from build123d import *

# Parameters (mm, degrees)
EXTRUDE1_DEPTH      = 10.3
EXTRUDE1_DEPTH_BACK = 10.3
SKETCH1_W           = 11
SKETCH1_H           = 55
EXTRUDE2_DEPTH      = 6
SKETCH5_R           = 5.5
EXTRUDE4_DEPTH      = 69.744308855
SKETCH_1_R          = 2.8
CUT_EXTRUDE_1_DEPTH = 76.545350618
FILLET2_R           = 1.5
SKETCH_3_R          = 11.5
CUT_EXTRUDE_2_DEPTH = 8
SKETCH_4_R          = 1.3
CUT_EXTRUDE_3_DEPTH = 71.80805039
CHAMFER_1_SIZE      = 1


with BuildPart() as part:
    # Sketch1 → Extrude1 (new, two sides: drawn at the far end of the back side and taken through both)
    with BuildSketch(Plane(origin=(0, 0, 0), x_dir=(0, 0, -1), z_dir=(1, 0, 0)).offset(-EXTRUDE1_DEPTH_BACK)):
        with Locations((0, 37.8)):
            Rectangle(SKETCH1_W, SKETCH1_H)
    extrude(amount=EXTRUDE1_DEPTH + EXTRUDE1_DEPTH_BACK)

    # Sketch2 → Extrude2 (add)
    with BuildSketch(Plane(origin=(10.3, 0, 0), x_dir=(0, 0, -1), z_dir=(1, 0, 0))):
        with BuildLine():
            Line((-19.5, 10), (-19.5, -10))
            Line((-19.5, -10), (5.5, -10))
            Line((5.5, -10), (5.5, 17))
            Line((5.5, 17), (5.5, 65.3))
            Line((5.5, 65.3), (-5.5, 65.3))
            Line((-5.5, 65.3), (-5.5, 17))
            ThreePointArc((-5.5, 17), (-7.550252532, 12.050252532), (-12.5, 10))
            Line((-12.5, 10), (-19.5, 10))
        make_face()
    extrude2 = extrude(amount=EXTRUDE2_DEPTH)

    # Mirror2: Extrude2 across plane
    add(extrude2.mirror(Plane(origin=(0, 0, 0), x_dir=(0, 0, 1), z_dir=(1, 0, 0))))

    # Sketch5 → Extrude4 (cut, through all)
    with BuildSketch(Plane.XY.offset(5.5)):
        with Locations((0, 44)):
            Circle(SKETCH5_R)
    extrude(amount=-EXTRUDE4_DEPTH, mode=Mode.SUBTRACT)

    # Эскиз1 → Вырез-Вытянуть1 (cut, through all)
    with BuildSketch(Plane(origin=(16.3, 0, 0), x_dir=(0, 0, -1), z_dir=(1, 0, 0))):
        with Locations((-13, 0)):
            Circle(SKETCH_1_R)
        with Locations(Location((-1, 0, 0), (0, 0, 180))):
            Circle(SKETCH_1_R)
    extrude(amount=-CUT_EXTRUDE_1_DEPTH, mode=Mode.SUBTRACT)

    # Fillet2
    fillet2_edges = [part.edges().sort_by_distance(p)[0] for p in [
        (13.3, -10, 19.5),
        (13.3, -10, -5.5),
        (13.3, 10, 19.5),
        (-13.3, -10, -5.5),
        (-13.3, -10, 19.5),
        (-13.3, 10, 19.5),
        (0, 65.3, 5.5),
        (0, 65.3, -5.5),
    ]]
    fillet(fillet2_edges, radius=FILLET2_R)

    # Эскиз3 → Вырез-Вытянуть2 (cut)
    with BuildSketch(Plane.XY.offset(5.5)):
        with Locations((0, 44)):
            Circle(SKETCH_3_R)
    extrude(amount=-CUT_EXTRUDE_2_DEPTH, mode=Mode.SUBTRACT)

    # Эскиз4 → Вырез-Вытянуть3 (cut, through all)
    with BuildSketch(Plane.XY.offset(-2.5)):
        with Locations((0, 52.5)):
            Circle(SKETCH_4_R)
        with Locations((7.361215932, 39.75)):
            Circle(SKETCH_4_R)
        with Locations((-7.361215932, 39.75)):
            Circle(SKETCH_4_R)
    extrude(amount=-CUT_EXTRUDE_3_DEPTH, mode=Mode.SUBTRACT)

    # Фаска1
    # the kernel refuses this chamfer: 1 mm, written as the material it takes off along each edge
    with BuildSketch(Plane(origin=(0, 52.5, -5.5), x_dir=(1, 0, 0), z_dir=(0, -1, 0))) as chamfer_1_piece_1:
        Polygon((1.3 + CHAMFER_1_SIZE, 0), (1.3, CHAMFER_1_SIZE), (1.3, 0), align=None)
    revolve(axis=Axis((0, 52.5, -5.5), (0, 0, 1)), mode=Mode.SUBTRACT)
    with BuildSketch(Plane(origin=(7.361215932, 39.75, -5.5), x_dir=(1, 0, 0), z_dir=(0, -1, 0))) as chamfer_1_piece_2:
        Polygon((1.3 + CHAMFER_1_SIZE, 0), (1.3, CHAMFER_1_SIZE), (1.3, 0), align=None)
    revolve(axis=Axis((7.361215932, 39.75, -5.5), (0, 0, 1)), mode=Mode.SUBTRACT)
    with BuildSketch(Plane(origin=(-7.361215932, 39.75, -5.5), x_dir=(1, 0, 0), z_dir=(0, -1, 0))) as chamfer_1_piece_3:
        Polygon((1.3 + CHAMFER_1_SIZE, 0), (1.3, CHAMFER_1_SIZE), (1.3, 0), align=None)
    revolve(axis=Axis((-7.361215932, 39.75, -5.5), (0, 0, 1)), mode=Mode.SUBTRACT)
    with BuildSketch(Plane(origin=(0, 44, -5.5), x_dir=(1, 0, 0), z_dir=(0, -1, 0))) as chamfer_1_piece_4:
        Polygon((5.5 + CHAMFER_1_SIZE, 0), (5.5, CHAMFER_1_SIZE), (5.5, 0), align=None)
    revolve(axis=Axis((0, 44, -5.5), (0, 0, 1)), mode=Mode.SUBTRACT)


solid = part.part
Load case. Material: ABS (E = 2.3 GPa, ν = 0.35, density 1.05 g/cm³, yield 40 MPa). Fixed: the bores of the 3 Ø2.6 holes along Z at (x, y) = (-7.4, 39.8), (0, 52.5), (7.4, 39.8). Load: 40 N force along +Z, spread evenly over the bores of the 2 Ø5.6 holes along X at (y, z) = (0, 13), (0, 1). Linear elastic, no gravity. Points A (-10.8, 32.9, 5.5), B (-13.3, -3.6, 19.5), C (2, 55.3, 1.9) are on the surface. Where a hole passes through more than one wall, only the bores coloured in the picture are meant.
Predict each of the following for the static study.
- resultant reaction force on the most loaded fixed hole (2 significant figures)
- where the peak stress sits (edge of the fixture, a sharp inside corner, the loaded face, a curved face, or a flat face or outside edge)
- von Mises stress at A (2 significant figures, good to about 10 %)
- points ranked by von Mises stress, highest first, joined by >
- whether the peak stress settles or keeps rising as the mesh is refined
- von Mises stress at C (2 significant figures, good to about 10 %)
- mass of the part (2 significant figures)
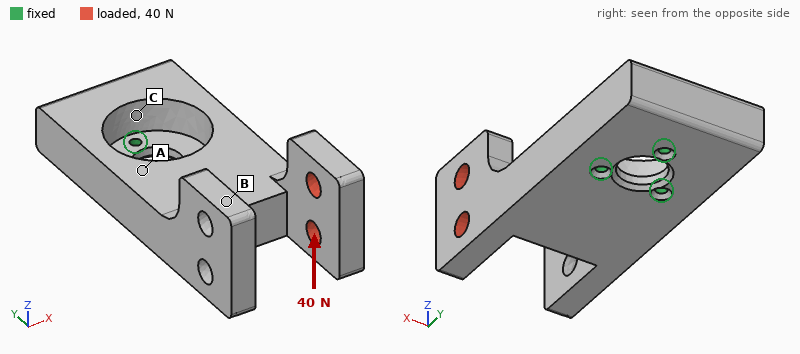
94 N
edge of the fixture
3.8 MPa
A > C > B
keeps rising
1.9 MPa
23 g
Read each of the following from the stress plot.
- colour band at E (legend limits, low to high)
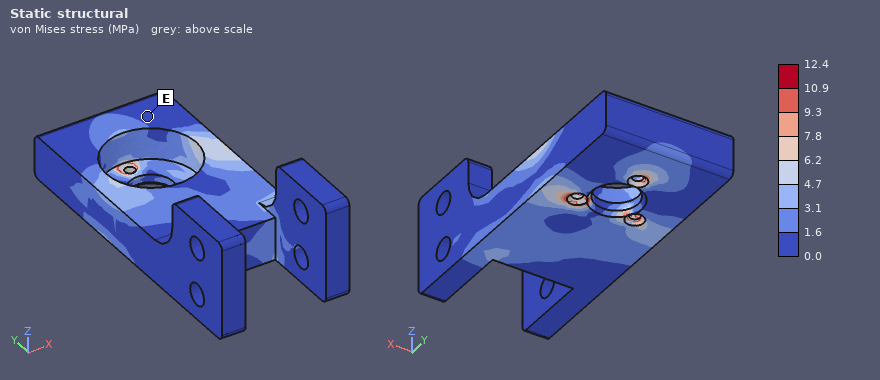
0.0 to 1.6 MPa
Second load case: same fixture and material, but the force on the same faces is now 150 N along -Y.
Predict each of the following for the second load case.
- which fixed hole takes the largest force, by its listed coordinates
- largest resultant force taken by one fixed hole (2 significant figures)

(7.4, 39.8)
150 N
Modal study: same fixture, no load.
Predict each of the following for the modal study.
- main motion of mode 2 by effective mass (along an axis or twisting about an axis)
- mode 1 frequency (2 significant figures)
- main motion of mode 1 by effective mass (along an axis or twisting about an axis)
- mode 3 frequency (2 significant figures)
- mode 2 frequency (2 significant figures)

along X
510 Hz
along Z
1300 Hz
1000 Hz
